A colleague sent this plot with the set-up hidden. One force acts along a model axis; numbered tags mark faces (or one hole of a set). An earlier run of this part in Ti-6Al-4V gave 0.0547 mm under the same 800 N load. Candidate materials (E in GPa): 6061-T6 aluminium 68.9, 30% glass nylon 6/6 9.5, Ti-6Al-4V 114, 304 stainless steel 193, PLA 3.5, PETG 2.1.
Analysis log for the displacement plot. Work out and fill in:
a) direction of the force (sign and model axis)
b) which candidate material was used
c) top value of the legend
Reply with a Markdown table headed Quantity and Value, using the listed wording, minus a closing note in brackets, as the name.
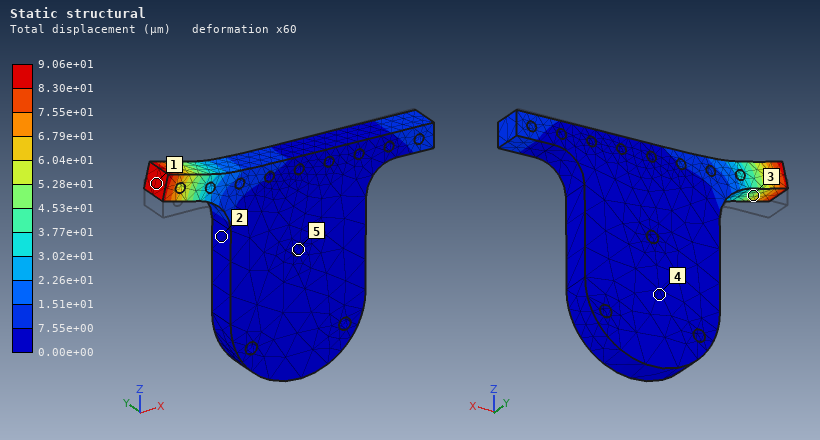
| Quantity | Value |
|---|---|
| direction of the force | +Z |
| which candidate material was used | 6061-T6 aluminium |
| top value of the legend | 9.06e+01 µm |
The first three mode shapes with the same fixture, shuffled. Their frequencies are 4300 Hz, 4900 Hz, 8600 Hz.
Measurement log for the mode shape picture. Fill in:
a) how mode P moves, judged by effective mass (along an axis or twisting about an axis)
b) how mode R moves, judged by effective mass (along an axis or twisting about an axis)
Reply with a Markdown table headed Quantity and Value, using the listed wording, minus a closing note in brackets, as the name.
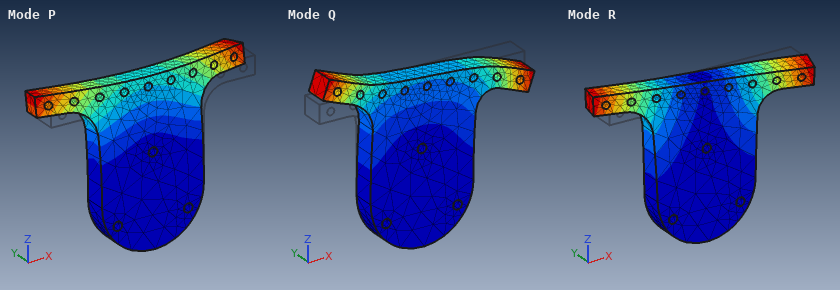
| Quantity | Value |
|---|---|
| how mode P moves, judged by effective mass | along Y |
| how mode R moves, judged by effective mass | twisting about Z |
